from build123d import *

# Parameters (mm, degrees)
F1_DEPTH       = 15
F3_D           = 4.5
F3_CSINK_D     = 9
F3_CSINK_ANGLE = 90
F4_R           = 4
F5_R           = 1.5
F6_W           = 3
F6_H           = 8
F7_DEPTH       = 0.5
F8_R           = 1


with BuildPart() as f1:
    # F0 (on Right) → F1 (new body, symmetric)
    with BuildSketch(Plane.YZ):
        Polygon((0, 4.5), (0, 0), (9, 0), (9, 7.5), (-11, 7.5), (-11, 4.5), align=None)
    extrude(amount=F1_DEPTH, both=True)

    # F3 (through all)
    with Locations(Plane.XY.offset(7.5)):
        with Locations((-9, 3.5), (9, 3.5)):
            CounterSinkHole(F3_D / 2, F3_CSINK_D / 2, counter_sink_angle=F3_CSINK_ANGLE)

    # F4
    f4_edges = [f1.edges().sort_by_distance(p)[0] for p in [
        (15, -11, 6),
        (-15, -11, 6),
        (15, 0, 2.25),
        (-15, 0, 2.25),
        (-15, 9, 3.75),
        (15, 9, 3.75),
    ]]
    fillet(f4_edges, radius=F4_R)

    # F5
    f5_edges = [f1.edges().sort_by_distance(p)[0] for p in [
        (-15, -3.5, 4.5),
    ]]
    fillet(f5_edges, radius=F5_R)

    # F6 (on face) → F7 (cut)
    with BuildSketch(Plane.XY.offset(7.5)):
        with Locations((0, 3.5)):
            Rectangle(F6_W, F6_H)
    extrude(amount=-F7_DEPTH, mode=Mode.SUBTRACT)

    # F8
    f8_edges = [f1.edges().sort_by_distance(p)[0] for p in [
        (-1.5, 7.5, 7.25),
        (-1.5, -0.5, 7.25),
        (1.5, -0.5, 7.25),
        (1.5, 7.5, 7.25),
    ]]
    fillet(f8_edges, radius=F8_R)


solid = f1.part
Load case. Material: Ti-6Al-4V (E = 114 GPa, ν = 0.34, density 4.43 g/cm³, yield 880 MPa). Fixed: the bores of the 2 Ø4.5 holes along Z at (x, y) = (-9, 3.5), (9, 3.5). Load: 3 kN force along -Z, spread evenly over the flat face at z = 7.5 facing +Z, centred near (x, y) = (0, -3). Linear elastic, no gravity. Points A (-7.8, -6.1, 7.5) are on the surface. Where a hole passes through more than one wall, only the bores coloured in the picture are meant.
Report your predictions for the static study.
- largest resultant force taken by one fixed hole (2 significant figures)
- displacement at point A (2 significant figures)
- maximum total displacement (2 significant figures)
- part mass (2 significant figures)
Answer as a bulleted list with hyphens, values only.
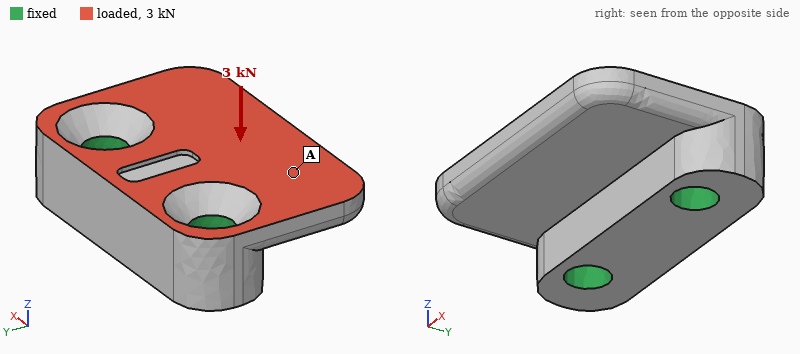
- 1.5 kN
- 0.068 mm
- 0.12 mm
- 11 g
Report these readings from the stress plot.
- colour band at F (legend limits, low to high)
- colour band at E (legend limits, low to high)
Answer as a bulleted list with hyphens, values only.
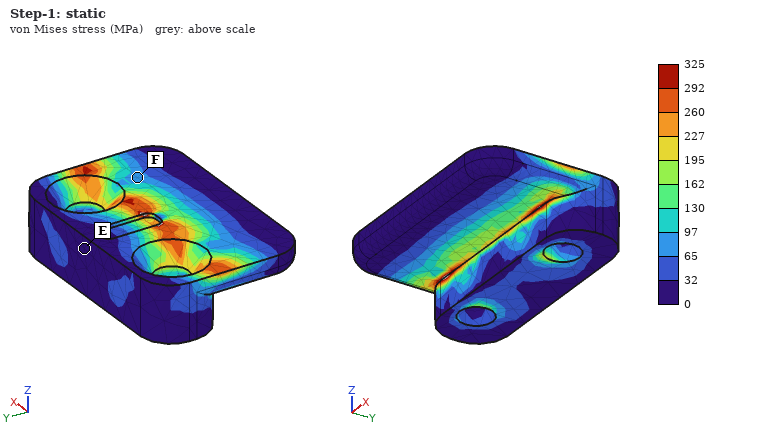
- 65 to 97 MPa
- 0 to 32 MPa
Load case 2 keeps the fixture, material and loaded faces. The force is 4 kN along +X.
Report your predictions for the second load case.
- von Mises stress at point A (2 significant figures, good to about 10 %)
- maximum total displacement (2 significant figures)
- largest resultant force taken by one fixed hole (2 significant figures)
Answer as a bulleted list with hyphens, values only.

- 59 MPa
- 21 µm
- 2.4 kN
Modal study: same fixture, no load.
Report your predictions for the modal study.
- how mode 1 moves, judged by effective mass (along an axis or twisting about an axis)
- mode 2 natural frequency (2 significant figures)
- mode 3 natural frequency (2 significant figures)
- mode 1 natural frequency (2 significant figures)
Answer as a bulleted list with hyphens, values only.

- along Z
- 19 kHz
- 33 kHz
- 13 kHz
